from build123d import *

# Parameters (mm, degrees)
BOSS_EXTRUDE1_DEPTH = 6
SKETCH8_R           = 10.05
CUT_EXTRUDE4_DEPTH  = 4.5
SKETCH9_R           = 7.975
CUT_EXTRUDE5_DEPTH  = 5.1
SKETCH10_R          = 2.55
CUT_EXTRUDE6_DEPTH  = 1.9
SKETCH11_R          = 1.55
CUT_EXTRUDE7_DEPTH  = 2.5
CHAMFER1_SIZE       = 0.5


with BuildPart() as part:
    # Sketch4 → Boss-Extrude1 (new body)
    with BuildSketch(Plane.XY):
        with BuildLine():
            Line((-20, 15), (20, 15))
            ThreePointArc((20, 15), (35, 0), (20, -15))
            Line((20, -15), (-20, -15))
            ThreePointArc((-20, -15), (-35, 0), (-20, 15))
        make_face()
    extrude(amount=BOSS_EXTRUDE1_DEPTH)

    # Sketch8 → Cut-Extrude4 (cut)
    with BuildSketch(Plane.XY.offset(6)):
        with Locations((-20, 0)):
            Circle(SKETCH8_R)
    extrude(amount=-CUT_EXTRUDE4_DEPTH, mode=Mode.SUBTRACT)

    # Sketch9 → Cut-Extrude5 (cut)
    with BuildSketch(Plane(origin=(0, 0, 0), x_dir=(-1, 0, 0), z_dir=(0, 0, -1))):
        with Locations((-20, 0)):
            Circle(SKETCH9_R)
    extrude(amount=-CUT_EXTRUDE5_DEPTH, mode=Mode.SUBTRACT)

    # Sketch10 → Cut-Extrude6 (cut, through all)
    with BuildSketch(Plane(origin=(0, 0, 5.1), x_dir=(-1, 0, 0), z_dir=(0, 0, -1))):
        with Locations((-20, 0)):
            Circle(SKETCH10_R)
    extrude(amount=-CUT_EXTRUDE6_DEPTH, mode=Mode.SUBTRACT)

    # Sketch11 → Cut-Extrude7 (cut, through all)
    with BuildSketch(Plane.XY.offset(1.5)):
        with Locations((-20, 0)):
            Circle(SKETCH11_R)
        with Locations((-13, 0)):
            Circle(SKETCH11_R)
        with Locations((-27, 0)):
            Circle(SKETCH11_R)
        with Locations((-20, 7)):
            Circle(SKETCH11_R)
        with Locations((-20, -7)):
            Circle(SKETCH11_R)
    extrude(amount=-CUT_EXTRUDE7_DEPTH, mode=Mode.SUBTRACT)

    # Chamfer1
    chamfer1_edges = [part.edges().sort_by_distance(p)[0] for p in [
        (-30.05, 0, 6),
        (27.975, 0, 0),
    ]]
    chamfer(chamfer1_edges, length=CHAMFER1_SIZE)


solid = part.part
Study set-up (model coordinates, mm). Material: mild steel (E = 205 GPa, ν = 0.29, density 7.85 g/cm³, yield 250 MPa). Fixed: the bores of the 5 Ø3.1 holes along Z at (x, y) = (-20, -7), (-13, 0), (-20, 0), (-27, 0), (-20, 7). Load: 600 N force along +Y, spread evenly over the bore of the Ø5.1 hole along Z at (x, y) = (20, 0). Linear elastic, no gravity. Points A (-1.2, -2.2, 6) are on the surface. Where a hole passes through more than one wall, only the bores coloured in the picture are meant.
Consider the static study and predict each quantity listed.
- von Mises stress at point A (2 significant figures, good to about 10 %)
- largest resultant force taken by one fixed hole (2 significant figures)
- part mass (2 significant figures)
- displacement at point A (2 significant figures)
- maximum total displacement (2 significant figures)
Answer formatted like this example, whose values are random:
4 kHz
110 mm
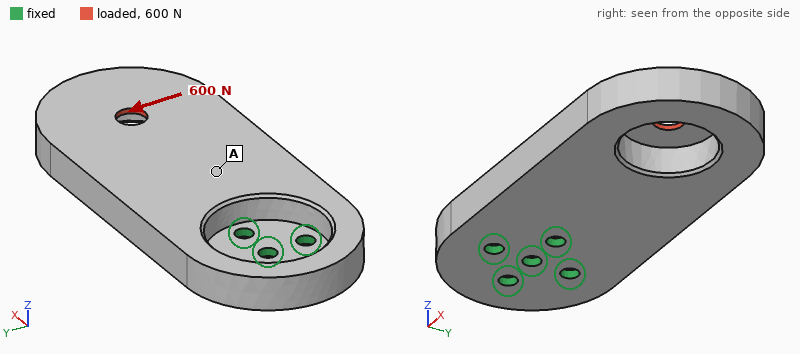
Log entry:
17 MPa
930 N
70 g
6.4 µm
21 µm
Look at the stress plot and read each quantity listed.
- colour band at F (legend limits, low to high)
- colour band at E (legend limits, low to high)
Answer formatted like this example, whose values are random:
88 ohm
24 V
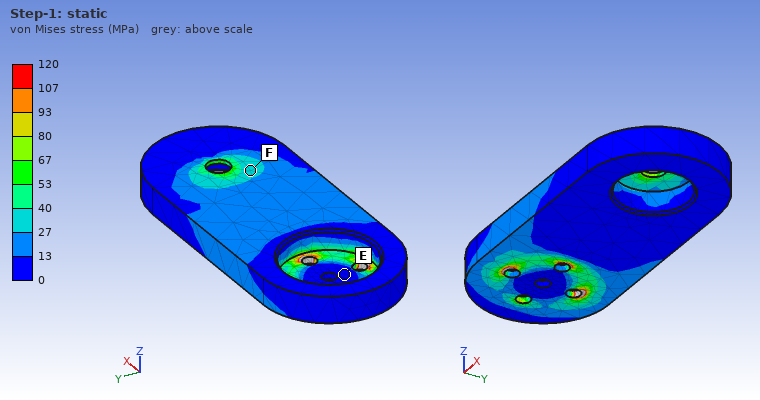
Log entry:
27 to 40 MPa
0 to 13 MPa
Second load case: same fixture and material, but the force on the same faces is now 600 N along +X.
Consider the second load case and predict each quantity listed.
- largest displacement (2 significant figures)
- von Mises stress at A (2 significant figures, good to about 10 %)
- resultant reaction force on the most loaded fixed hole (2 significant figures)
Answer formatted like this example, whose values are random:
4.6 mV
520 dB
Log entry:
38 µm
8.2 MPa
260 N
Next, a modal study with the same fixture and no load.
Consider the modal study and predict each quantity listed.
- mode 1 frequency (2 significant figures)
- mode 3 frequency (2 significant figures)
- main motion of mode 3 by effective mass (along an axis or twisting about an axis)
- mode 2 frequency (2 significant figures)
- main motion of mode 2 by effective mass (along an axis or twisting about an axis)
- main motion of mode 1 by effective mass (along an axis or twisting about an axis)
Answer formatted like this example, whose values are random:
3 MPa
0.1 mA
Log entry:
1600 Hz
5700 Hz
along Y
4900 Hz
twisting about X
along Z
